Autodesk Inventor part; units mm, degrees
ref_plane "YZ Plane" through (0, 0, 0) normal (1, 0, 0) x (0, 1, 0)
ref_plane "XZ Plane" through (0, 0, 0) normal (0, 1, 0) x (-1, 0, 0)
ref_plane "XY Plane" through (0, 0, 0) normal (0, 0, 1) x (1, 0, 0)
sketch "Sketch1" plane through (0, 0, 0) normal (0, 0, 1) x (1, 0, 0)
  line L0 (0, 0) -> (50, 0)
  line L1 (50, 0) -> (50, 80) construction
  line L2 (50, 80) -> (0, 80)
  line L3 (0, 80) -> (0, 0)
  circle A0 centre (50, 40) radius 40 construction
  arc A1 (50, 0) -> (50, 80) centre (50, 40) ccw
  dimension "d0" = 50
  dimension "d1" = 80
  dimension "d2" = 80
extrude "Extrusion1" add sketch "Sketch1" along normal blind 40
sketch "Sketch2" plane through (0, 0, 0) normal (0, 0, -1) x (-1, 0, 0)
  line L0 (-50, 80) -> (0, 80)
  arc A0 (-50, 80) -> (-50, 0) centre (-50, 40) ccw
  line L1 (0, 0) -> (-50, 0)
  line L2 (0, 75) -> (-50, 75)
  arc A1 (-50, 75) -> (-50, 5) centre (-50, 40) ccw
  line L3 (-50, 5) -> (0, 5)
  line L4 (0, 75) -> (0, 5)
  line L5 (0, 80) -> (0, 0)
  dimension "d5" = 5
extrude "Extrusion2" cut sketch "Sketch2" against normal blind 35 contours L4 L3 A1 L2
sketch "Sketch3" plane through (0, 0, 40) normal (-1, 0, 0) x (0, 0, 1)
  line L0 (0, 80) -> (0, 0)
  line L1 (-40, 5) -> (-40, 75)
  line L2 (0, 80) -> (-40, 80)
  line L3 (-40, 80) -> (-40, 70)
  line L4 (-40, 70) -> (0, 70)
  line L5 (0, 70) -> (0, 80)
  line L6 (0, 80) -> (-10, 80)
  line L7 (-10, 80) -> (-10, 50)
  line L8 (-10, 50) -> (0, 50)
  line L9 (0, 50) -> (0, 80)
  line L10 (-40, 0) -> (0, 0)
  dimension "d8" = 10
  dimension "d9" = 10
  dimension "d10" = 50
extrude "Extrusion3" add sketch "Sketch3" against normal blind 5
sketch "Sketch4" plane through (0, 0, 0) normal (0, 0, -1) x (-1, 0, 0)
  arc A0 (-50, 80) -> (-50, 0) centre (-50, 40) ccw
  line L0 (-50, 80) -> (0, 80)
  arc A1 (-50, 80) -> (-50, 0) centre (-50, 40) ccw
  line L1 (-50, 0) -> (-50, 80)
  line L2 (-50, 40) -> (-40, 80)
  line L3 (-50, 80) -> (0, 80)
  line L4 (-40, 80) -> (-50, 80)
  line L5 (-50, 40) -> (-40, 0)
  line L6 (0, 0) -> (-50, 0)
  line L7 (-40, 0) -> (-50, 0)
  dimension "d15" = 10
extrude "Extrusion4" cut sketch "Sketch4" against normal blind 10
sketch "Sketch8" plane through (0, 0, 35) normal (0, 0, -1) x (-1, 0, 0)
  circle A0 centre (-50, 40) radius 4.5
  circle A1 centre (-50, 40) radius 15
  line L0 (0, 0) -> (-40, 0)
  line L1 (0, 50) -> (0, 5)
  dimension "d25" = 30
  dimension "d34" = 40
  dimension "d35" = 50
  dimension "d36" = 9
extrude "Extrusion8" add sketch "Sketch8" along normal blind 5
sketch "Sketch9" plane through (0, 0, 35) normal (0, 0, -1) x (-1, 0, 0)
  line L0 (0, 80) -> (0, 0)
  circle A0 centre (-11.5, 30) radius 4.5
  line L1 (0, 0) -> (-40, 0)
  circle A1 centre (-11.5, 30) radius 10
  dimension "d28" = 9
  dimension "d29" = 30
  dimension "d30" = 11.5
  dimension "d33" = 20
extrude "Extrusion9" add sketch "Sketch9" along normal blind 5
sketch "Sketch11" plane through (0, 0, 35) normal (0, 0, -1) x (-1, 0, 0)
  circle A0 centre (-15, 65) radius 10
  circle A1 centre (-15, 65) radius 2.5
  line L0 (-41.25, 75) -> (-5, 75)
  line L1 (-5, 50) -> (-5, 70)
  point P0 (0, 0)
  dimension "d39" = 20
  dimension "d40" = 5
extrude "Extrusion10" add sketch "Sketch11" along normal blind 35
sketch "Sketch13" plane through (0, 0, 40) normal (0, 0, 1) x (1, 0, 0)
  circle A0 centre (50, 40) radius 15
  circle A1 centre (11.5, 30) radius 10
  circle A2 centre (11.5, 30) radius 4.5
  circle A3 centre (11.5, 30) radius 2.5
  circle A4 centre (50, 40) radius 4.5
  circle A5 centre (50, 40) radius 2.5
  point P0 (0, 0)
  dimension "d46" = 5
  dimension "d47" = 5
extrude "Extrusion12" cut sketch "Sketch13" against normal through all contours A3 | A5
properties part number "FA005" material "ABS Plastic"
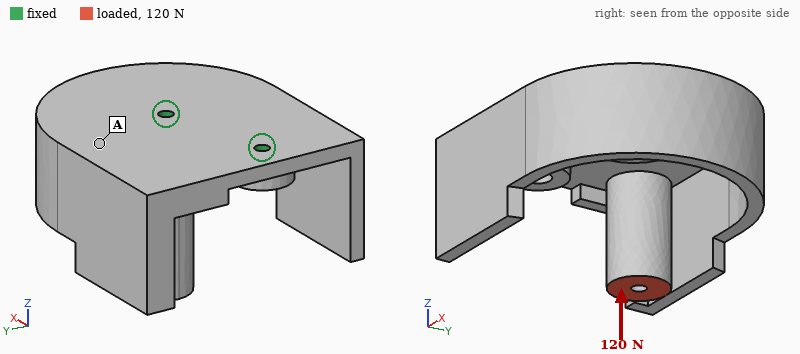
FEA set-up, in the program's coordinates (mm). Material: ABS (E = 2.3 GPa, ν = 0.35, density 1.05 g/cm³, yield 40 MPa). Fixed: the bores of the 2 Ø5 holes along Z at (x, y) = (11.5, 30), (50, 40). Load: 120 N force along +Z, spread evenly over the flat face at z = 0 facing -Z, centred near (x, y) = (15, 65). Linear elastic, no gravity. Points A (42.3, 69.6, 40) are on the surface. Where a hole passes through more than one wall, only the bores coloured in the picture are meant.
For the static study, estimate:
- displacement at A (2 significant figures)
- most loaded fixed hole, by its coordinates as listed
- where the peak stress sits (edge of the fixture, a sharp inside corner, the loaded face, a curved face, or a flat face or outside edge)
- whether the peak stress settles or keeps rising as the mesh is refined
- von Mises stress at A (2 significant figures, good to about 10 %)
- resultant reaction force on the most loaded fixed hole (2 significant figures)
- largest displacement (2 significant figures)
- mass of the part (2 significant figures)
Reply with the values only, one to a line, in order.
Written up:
0.45 mm
(11.5, 30)
edge of the fixture
keeps rising
1.6 MPa
81 N
1.4 mm
84 g
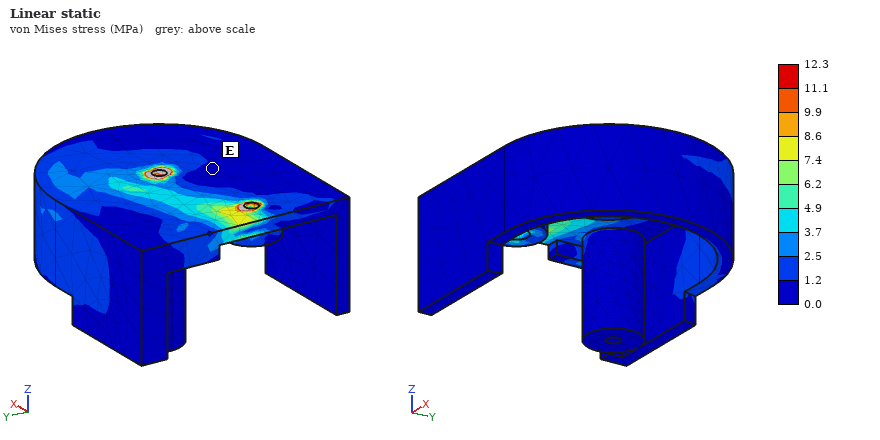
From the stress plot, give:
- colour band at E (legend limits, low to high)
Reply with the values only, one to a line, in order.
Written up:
0.0 to 1.2 MPa
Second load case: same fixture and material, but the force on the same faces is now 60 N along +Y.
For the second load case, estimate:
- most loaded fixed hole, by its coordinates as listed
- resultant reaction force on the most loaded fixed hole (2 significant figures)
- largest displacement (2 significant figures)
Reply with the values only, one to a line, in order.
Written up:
(11.5, 30)
56 N
1.3 mm
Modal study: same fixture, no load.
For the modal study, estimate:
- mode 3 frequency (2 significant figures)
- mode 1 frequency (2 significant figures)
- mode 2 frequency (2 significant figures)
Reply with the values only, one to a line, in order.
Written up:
670 Hz
270 Hz
460 Hz
